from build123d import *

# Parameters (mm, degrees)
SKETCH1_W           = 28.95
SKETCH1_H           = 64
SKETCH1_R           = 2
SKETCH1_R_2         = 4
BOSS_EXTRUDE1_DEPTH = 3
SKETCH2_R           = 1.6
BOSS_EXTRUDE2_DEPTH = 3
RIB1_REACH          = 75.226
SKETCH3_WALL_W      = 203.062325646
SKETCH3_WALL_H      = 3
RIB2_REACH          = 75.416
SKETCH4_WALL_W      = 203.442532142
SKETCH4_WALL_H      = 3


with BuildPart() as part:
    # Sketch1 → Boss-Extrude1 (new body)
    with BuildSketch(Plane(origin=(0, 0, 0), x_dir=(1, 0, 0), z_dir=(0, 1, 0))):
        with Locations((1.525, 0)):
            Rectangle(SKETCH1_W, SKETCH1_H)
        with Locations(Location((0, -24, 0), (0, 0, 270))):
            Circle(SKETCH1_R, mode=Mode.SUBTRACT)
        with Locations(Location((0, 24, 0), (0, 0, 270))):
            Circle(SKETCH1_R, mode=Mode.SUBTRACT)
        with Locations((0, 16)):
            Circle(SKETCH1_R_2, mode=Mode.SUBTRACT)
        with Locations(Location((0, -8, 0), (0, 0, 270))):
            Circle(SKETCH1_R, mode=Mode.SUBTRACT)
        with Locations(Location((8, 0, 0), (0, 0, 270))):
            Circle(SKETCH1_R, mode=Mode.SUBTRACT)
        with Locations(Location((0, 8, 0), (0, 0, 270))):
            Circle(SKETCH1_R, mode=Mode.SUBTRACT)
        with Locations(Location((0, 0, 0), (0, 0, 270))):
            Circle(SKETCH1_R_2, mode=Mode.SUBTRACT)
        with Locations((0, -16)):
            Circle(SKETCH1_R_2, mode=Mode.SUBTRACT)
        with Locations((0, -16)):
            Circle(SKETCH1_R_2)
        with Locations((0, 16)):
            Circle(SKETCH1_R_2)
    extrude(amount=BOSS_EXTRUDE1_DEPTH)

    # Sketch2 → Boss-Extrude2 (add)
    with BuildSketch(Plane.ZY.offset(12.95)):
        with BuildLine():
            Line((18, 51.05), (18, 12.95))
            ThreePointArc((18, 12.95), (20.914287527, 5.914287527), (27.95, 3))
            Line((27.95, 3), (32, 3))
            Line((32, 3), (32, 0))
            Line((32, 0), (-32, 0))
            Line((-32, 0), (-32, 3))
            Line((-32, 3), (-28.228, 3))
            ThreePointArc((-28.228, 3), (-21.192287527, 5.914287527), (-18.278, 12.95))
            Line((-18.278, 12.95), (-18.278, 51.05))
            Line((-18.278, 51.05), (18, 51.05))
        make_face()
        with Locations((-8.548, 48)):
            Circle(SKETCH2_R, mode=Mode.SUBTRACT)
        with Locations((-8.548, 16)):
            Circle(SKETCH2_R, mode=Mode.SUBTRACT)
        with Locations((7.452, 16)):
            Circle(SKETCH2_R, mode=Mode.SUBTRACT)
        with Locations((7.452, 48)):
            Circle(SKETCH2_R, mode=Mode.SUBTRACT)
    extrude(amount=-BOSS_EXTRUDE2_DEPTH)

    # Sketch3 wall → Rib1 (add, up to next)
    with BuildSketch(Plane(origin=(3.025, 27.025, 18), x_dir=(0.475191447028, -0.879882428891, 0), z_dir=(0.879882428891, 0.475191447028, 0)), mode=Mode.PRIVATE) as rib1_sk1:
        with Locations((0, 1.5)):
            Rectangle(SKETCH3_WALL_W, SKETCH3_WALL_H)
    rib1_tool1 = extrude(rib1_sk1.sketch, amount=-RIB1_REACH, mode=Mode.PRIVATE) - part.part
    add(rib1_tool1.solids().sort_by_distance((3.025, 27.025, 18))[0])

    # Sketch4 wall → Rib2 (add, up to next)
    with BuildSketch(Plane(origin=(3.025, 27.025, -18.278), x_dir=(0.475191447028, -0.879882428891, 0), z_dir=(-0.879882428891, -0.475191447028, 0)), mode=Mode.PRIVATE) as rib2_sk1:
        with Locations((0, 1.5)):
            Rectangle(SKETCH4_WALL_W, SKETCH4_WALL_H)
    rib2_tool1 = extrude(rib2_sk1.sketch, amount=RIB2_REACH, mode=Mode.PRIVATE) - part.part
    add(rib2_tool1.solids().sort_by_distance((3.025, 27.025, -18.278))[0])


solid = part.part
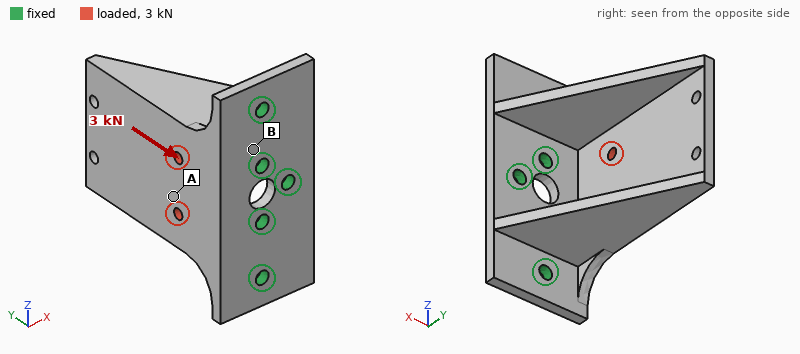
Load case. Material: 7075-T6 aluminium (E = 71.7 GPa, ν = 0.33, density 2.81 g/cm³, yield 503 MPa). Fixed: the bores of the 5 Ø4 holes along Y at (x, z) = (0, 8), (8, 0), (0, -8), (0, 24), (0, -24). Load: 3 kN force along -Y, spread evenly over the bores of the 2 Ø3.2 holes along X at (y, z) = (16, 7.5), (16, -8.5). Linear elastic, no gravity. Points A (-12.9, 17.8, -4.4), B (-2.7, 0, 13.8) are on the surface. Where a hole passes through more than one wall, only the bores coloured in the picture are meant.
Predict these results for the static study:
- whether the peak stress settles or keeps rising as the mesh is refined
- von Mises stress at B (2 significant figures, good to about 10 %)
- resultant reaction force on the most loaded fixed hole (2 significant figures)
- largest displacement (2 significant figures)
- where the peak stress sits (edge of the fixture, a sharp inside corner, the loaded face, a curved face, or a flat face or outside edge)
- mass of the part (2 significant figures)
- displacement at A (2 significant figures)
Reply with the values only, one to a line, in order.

keeps rising
80 MPa
1.1 kN
0.30 mm
edge of the fixture
40 g
0.13 mm
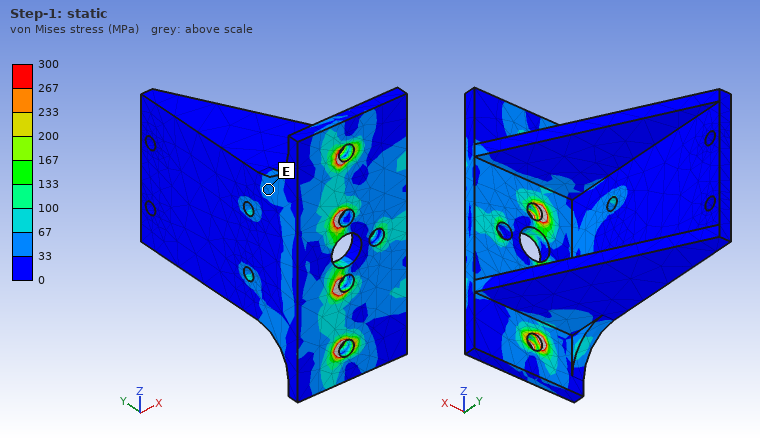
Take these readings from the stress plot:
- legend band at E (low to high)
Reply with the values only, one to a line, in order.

33 to 67 MPa
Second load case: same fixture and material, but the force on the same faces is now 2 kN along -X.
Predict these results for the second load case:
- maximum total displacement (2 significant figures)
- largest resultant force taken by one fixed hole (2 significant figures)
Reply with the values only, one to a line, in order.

0.29 mm
740 N
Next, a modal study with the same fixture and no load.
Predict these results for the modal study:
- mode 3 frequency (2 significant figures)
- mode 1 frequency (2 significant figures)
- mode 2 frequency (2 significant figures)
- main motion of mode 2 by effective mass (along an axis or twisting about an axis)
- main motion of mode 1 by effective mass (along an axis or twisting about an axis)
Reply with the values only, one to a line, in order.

8600 Hz
2600 Hz
3500 Hz
along Z
along X
